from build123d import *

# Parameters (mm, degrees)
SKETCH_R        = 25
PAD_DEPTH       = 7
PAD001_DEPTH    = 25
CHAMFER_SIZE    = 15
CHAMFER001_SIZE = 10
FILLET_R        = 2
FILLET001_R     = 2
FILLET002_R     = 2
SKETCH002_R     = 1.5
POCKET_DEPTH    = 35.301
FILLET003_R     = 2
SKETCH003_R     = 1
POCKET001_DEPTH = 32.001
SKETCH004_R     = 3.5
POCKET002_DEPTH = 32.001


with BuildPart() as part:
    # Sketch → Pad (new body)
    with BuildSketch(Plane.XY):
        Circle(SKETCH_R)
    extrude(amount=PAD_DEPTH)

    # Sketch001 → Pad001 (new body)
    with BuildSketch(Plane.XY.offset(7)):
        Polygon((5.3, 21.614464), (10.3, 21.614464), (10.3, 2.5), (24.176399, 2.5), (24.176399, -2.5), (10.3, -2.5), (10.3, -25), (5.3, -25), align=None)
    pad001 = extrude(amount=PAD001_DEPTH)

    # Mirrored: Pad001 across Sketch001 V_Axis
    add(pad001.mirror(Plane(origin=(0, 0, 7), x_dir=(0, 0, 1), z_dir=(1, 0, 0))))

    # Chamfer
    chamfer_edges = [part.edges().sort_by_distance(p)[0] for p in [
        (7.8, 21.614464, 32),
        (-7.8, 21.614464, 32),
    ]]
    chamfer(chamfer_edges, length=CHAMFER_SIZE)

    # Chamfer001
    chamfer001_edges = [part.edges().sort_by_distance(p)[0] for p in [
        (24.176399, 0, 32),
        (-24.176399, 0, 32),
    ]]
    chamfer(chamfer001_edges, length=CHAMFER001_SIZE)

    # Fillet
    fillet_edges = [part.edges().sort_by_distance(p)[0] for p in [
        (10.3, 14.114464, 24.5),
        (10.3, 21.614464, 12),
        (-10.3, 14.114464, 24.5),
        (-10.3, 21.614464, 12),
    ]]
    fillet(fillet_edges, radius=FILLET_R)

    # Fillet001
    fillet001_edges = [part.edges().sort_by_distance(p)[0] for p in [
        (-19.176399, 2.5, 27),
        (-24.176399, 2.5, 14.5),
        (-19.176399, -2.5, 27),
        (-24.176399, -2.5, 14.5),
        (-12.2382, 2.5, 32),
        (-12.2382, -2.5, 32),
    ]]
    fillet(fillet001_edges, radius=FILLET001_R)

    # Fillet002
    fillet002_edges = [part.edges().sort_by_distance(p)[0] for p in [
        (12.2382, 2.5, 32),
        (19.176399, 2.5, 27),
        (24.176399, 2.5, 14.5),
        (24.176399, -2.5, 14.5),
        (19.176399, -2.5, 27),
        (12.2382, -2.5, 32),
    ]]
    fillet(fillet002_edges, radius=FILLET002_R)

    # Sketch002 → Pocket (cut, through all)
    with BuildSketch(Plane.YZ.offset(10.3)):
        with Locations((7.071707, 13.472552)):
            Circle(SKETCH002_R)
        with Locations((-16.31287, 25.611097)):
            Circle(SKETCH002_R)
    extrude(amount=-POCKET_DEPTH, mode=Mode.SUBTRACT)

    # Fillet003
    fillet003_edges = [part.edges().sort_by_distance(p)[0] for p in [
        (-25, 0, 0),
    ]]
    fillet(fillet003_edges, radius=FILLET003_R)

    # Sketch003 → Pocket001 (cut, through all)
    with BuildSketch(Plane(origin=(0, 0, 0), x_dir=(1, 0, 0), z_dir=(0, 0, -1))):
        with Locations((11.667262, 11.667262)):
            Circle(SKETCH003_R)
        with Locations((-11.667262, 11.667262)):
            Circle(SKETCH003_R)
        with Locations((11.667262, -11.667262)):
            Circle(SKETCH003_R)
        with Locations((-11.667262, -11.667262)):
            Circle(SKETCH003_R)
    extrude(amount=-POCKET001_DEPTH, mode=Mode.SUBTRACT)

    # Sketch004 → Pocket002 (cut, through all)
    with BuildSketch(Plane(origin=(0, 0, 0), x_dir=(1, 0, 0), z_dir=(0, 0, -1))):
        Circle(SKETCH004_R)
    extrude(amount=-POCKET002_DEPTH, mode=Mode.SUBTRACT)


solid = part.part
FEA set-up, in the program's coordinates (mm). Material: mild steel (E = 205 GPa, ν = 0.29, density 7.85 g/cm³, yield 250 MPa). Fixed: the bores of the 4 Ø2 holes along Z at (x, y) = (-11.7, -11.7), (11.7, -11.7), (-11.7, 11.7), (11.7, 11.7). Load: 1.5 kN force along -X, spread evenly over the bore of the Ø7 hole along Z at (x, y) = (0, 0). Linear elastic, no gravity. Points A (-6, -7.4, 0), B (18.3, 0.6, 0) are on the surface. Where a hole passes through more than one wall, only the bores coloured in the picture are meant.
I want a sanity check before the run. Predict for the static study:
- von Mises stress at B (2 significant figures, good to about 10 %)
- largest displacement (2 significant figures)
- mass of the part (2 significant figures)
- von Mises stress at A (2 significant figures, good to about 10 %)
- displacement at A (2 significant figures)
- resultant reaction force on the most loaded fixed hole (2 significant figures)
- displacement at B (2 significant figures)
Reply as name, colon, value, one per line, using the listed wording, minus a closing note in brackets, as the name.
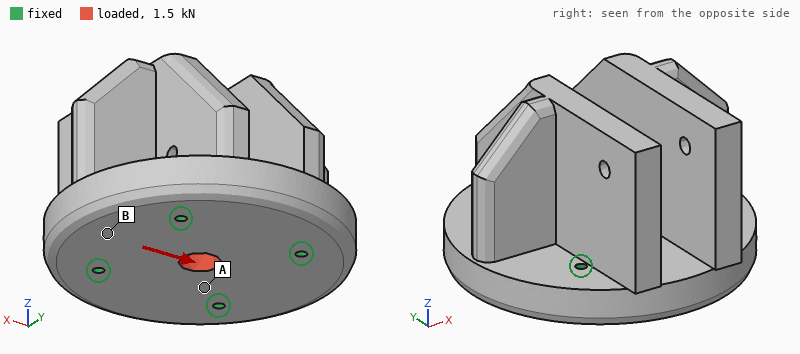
von Mises stress at B: 1.9 MPa
largest displacement: 0.59 µm
mass of the part: 210 g
von Mises stress at A: 6.1 MPa
displacement at A: 0.24 µm
resultant reaction force on the most loaded fixed hole: 390 N
displacement at B: 0.25 µm
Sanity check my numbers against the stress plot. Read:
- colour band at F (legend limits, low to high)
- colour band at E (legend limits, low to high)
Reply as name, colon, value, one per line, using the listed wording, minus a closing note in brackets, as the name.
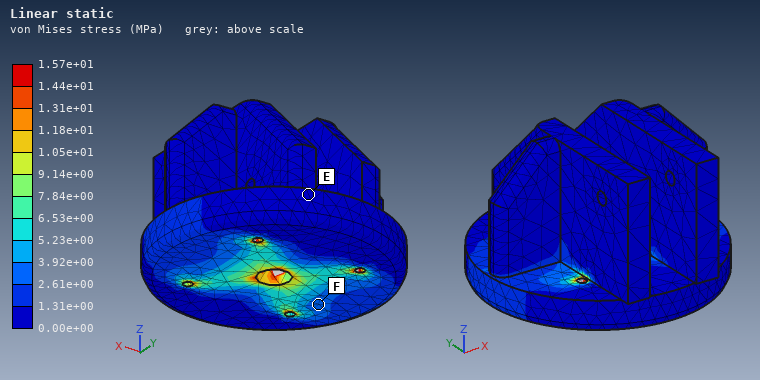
colour band at F: 2.61e+00 to 3.92e+00 MPa
colour band at E: 0.00e+00 to 1.31e+00 MPa
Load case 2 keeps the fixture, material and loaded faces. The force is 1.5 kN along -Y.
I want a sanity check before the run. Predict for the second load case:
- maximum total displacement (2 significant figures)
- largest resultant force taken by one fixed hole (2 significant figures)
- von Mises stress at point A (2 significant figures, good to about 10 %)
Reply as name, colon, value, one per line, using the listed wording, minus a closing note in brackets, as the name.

maximum total displacement: 0.57 µm
largest resultant force taken by one fixed hole: 390 N
von Mises stress at point A: 6.1 MPa
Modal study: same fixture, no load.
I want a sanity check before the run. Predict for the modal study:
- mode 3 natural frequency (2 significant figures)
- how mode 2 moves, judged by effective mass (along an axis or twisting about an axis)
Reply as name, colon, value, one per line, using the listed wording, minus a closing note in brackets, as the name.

mode 3 natural frequency: 11 kHz
how mode 2 moves, judged by effective mass: along X
